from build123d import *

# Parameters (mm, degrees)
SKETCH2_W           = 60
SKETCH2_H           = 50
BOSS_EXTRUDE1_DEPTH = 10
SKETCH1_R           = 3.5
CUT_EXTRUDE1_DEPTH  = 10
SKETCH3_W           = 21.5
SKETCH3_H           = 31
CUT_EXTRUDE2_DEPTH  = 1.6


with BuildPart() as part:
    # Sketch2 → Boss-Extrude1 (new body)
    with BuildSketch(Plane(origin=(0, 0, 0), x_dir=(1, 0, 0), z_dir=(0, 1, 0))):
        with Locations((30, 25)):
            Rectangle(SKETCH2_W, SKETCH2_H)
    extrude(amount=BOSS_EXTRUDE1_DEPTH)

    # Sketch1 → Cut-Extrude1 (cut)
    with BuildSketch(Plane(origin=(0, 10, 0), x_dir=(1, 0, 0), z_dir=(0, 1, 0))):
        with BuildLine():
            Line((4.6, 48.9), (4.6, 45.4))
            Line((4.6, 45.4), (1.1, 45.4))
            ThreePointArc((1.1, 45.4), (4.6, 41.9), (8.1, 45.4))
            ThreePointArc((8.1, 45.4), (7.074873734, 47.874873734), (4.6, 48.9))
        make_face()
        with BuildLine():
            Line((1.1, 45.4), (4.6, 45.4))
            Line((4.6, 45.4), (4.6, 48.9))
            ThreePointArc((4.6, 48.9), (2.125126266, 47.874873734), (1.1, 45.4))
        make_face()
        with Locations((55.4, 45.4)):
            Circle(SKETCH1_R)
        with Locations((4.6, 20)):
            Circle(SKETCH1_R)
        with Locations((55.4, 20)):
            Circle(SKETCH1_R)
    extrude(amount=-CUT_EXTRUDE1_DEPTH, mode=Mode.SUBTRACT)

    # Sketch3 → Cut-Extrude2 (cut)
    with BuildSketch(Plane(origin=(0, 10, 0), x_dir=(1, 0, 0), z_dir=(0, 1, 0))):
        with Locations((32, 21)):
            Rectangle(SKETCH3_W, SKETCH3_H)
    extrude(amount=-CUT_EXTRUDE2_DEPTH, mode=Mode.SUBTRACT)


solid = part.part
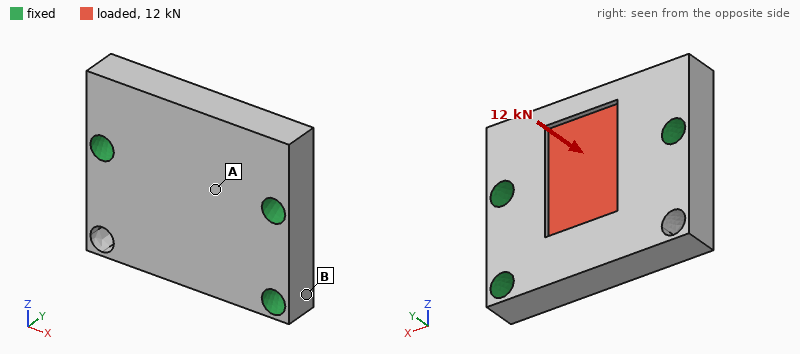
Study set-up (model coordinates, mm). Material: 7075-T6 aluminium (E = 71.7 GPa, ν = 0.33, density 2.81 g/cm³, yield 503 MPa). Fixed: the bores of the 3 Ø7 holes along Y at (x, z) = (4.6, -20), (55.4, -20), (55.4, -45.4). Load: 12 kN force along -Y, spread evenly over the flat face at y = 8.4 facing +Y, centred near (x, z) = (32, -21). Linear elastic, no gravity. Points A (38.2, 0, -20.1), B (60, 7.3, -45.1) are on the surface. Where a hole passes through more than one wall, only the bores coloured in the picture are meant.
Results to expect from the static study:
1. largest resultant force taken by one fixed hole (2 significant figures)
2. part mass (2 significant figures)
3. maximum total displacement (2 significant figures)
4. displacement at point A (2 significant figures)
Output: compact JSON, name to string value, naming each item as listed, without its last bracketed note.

{"largest resultant force taken by one fixed hole": "5.6 kN", "part mass": "77 g", "maximum total displacement": "63 µm", "displacement at point A": "42 µm"}
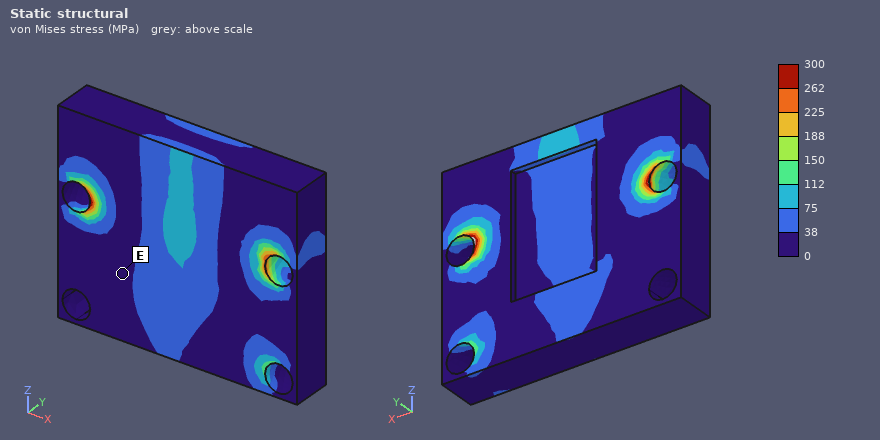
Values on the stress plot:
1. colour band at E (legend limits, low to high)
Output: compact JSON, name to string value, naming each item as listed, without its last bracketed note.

{"colour band at E": "0 to 38 MPa"}
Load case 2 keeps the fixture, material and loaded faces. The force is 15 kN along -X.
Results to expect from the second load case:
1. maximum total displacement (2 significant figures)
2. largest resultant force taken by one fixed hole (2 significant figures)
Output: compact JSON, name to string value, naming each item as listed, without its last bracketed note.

{"maximum total displacement": "13 µm", "largest resultant force taken by one fixed hole": "6.5 kN"}
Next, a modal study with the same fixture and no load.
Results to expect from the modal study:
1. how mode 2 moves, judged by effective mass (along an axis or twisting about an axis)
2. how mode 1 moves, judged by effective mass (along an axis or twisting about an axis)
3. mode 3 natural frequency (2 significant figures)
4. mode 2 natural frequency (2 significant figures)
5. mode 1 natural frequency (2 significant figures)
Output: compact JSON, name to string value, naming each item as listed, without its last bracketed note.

{"how mode 2 moves, judged by effective mass": "along Y", "how mode 1 moves, judged by effective mass": "along Y", "mode 3 natural frequency": "20 kHz", "mode 2 natural frequency": "13 kHz", "mode 1 natural frequency": "10 kHz"}
